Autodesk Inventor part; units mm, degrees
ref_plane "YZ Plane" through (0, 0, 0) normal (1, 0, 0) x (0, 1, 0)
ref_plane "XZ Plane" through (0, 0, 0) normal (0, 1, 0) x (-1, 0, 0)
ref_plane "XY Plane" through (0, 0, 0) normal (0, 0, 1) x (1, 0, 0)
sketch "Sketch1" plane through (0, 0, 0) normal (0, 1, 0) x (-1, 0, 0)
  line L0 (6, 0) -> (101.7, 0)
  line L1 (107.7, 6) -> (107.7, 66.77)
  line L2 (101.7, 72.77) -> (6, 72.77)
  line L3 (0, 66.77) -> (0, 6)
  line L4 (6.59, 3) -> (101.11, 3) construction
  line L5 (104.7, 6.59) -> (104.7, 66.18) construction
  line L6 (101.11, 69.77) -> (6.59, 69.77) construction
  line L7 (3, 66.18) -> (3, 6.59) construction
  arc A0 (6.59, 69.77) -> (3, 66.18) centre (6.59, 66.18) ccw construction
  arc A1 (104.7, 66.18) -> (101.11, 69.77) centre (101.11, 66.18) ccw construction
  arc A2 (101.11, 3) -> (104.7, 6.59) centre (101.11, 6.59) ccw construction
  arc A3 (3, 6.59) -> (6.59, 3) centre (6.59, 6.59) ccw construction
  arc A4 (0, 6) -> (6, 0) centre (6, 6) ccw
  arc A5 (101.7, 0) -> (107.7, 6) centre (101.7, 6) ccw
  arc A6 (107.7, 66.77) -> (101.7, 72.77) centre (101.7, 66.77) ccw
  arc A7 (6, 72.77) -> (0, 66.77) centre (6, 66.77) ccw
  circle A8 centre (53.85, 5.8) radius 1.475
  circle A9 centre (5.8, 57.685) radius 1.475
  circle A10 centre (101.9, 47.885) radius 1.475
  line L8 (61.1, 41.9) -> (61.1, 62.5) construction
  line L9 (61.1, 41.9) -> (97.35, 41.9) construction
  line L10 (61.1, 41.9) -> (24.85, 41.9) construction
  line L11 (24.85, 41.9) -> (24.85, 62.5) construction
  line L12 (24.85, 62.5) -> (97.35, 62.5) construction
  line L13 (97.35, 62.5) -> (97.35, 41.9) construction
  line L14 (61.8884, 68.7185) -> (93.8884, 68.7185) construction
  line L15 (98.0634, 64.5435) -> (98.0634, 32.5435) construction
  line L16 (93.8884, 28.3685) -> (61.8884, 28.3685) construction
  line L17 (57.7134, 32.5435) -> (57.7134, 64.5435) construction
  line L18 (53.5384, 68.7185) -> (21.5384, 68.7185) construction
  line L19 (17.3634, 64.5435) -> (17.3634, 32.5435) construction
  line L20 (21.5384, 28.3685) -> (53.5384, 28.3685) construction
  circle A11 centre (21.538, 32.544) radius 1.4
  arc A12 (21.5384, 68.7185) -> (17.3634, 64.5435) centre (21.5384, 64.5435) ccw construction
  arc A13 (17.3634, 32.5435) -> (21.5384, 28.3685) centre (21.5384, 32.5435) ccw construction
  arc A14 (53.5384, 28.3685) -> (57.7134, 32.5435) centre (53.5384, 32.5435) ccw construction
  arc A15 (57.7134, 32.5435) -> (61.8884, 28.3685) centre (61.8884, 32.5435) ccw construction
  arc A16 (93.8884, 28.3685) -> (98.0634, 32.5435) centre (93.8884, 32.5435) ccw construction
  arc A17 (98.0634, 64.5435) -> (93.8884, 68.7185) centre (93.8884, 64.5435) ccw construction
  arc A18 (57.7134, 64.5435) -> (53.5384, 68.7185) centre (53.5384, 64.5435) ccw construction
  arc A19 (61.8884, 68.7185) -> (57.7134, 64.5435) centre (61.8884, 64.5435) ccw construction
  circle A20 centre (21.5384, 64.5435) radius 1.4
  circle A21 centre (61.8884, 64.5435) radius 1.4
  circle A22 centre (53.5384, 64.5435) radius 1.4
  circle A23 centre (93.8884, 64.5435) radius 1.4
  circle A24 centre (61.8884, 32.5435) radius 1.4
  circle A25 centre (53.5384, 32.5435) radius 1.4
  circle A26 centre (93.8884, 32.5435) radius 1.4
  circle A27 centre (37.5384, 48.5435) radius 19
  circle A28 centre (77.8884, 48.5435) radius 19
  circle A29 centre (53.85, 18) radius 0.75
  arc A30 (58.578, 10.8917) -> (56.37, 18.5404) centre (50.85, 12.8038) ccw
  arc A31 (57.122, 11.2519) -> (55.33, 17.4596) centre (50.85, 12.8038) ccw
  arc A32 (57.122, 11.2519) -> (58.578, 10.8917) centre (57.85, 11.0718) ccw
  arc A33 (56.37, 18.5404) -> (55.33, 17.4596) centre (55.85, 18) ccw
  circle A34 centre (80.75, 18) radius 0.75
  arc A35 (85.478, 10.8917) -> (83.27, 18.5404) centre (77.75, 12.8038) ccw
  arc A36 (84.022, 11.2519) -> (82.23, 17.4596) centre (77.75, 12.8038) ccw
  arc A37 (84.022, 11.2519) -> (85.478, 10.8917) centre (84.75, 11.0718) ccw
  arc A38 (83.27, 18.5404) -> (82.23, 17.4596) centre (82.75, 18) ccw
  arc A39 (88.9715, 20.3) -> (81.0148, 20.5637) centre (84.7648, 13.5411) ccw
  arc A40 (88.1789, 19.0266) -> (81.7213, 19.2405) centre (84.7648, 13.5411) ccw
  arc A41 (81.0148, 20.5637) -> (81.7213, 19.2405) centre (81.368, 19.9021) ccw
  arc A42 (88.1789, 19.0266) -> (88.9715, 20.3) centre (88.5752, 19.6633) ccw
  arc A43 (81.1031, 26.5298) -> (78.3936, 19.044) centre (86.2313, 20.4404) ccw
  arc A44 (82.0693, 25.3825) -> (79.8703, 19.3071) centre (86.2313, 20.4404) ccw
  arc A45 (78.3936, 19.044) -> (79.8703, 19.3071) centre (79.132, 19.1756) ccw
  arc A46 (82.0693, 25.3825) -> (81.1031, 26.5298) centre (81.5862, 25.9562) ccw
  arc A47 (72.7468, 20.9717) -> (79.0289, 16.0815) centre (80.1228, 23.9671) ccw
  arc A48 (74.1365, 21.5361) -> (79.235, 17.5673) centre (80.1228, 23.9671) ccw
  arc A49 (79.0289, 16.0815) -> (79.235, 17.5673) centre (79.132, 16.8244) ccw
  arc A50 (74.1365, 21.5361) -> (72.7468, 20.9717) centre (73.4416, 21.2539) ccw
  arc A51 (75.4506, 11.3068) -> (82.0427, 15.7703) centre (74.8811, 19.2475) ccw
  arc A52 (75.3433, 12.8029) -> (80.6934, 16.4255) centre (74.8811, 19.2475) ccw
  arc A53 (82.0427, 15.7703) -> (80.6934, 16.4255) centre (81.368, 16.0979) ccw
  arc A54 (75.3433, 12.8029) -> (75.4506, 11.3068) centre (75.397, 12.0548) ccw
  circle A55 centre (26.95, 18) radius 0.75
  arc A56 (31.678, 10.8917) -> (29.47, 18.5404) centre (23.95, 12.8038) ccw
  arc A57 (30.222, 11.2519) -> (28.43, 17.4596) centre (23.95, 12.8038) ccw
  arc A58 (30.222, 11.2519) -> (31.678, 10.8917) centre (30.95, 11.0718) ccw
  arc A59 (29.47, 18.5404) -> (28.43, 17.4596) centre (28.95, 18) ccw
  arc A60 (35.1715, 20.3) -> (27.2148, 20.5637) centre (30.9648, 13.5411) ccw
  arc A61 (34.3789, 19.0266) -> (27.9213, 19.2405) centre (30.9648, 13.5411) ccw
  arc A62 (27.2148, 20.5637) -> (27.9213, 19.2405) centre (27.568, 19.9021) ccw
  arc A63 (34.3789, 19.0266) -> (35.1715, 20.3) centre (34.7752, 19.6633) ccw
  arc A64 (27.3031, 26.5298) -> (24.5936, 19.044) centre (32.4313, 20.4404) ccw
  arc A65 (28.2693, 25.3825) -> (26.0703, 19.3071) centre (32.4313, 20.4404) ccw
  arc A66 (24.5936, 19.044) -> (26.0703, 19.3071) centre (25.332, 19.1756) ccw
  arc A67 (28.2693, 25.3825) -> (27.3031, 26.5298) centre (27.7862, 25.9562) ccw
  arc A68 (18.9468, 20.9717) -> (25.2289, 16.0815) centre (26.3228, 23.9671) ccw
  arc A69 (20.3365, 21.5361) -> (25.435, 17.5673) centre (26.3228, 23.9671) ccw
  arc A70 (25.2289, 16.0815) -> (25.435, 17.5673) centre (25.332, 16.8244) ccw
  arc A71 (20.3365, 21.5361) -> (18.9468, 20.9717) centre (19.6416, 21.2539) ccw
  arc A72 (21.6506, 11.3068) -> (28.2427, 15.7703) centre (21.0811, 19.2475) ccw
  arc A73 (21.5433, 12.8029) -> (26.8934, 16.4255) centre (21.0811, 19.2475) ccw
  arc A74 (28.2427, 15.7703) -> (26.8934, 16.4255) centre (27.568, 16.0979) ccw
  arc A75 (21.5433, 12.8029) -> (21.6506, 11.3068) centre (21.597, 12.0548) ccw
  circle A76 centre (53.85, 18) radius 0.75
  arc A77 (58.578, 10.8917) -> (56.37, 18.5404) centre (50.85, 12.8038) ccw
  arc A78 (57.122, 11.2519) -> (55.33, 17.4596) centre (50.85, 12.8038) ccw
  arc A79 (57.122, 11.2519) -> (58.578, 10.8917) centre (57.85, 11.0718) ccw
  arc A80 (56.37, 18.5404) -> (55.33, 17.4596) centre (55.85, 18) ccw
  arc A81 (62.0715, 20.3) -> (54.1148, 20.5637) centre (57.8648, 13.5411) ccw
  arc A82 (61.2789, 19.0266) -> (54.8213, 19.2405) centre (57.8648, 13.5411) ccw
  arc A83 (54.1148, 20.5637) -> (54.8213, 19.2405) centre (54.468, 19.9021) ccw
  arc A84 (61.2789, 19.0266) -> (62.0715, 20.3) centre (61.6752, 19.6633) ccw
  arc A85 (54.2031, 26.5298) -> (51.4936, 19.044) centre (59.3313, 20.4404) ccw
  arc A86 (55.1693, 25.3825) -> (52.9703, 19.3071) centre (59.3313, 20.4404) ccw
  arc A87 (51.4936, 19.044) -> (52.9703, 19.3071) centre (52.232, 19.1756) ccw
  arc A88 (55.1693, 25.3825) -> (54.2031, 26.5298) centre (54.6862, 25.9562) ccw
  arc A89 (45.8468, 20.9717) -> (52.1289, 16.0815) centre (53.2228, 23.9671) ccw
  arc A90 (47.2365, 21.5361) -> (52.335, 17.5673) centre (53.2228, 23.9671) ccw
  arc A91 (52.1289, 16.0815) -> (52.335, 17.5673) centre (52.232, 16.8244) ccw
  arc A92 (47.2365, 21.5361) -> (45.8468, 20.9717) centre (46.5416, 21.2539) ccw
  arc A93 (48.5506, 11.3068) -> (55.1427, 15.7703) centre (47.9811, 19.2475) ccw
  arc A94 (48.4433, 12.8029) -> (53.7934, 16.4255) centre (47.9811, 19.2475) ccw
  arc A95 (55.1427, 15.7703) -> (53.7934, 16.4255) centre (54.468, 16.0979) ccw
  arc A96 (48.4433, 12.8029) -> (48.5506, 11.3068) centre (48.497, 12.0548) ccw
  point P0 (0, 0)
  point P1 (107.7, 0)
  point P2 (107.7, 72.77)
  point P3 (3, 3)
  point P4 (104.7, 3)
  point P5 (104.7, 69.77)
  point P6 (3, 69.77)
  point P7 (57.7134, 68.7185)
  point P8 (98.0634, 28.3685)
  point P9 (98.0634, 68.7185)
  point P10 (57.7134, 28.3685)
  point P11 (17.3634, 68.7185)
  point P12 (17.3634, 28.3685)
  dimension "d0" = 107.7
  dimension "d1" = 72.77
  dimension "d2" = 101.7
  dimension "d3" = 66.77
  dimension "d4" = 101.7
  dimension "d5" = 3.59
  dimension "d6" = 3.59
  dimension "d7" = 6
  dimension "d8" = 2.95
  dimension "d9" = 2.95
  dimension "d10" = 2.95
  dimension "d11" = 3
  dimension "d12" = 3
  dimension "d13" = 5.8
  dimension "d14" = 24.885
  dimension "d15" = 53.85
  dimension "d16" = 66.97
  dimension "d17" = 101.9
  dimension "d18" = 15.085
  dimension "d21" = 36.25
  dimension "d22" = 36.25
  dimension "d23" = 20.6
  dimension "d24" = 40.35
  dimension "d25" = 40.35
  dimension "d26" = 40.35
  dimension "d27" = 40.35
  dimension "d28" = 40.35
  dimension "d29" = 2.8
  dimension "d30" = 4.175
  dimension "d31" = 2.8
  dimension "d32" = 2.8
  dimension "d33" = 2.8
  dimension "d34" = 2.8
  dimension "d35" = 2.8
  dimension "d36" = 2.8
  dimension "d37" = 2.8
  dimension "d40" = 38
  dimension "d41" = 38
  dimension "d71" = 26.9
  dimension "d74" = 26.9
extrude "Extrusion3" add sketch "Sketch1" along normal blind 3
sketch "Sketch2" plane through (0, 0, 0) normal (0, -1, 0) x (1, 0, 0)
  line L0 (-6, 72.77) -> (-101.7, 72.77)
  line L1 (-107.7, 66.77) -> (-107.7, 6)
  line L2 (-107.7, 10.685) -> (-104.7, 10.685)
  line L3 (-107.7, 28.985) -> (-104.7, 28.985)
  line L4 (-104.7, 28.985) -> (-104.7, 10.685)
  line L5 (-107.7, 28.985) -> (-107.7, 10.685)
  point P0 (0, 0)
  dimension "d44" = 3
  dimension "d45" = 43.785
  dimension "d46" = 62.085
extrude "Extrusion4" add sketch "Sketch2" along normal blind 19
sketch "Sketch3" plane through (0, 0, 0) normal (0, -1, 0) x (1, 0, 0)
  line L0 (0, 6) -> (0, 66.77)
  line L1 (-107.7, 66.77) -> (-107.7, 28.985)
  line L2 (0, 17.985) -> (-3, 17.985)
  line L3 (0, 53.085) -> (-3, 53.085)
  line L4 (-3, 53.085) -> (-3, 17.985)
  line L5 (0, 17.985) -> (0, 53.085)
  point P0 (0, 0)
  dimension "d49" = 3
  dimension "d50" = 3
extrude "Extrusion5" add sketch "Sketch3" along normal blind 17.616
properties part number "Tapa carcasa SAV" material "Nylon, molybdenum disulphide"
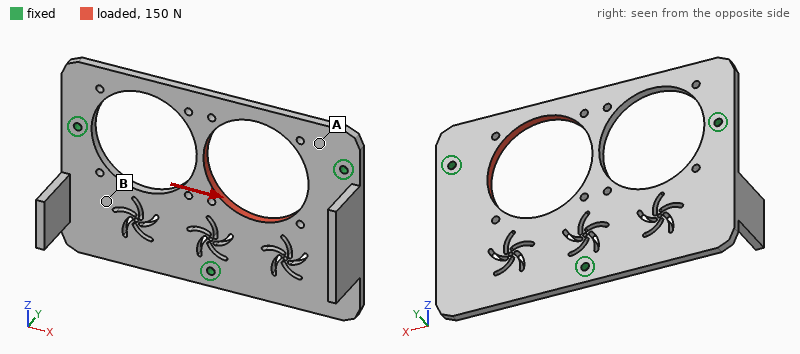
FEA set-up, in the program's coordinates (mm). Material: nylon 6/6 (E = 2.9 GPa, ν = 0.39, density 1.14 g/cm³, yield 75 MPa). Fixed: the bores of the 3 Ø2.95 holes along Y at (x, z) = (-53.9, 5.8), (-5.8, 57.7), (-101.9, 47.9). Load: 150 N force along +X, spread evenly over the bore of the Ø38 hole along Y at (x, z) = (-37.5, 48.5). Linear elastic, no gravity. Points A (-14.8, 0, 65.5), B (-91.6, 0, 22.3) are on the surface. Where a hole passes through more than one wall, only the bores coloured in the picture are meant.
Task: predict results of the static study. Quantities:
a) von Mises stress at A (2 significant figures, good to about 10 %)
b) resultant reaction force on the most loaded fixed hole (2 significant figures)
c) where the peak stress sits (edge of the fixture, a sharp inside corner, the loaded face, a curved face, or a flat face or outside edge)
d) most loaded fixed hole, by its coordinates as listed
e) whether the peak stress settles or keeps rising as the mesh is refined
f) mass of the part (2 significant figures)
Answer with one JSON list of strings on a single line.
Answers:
["1.8 MPa", "89 N", "edge of the fixture", "(-5.8, 57.7)", "keeps rising", "21 g"]
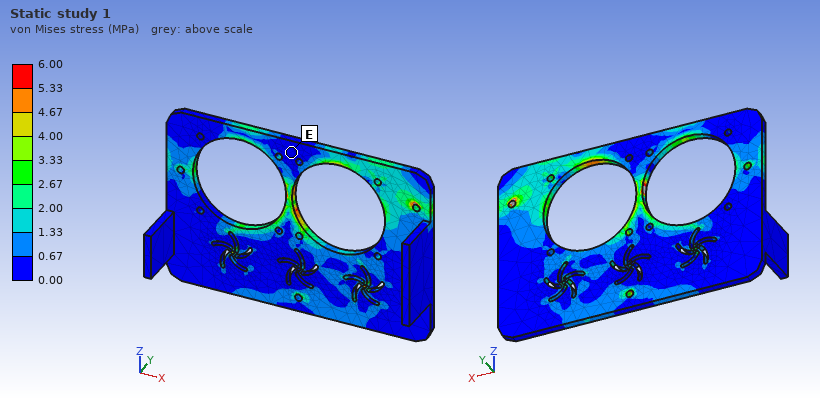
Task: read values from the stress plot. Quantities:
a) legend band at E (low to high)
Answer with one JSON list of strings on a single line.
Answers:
["0.00 to 0.67 MPa"]
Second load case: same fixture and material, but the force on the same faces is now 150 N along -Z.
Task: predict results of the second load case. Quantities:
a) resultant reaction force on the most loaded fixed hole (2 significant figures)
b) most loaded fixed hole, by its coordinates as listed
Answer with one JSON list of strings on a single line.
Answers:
["79 N", "(-5.8, 57.7)"]
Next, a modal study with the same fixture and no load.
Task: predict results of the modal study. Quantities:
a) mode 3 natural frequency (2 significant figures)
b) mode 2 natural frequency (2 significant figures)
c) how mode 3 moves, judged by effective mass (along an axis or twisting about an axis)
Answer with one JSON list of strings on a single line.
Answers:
["500 Hz", "400 Hz", "along Y"]
